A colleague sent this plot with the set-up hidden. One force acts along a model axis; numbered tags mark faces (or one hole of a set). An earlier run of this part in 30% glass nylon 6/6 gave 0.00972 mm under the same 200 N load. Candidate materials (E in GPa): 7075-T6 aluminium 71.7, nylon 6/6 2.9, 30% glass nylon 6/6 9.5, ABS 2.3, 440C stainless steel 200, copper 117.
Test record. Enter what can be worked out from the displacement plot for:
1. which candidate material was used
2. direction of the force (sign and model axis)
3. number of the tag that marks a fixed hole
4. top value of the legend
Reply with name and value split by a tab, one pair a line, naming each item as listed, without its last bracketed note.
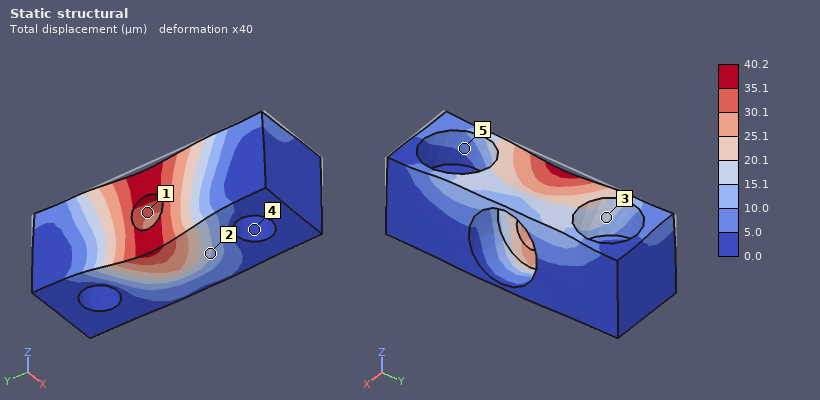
which candidate material was used	ABS
direction of the force	-Z
number of the tag that marks a fixed hole	4
top value of the legend	40.2 µm
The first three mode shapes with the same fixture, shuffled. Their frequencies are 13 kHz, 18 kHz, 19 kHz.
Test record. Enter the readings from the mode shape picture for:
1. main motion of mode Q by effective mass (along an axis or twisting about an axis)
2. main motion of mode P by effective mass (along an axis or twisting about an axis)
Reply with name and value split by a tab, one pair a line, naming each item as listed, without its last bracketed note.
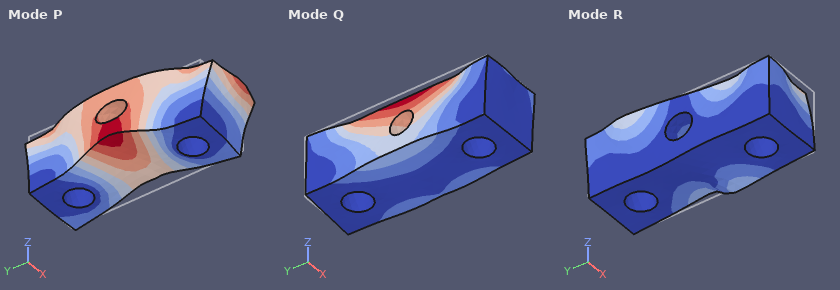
main motion of mode Q by effective mass	along X
main motion of mode P by effective mass	along Z
